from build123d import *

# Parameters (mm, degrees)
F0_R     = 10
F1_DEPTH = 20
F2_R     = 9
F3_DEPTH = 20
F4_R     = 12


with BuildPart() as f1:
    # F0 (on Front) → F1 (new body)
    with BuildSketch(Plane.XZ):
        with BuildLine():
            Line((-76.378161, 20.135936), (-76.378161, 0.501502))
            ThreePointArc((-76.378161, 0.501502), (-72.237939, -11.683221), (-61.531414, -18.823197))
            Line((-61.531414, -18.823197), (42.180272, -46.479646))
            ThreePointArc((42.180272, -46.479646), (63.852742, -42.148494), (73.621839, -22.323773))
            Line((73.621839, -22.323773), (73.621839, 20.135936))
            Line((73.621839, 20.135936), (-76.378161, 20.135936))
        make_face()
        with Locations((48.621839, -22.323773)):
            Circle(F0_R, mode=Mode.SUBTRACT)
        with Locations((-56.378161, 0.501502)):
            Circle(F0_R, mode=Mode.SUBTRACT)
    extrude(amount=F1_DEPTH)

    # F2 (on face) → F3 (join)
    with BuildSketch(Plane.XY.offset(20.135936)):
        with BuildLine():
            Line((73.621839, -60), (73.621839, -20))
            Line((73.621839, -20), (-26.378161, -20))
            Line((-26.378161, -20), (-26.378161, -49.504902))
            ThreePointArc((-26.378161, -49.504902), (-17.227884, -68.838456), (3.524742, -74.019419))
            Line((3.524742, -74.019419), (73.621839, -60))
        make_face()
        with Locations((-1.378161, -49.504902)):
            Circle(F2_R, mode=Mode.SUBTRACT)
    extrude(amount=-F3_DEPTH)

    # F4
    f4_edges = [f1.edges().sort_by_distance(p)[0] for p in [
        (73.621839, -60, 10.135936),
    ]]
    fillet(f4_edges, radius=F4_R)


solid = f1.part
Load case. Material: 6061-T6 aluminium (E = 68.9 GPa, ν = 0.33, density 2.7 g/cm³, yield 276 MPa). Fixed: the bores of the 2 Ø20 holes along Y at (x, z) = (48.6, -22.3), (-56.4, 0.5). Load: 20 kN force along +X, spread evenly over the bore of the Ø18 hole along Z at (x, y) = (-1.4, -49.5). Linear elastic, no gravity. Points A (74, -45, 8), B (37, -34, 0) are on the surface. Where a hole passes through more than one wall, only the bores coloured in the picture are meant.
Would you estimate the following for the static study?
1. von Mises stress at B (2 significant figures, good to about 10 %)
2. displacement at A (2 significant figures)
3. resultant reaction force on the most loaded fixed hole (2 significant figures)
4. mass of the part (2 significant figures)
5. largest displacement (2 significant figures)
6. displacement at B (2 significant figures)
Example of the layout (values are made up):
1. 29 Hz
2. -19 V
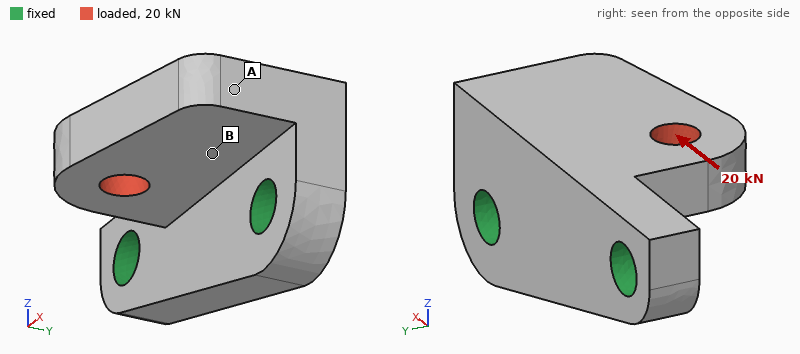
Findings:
1. 24 MPa
2. 66 µm
3. 13 kN
4. 640 g
5. 81 µm
6. 37 µm
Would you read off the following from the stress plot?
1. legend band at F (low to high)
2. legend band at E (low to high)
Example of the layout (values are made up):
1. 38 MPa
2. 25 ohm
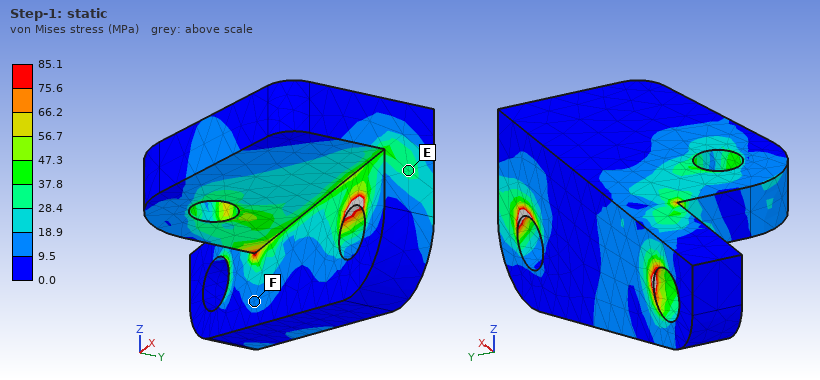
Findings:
1. 9.5 to 18.9 MPa
2. 28.4 to 37.8 MPa
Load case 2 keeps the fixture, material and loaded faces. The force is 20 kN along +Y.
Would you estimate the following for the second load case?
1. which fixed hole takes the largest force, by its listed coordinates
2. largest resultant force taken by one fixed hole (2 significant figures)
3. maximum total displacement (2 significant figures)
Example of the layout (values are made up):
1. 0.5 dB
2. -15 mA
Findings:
1. (-56.4, 0.5)
2. 11 kN
3. 0.13 mm
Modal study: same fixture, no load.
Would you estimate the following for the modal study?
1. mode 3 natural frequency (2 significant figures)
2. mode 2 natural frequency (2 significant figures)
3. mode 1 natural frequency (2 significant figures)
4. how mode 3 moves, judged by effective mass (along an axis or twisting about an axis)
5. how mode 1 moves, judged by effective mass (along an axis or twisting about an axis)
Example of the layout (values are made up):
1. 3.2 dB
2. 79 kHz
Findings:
1. 6500 Hz
2. 5600 Hz
3. 2900 Hz
4. along Y
5. along Z
